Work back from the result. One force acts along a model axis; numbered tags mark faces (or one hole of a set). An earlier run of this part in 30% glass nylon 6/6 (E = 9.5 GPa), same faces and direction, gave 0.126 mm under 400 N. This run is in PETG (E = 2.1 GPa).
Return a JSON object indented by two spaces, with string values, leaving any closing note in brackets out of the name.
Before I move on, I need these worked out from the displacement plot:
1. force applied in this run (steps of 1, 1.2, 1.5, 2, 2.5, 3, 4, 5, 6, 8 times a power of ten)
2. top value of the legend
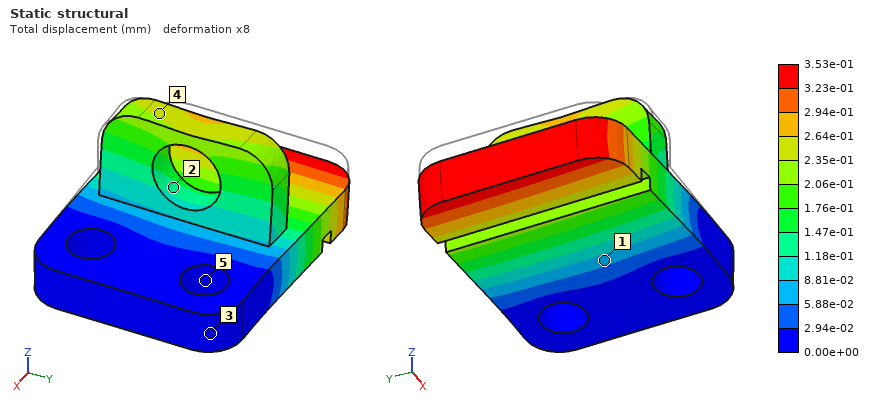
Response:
{
  "force applied in this run": "250 N",
  "top value of the legend": "3.53e-01 mm"
}
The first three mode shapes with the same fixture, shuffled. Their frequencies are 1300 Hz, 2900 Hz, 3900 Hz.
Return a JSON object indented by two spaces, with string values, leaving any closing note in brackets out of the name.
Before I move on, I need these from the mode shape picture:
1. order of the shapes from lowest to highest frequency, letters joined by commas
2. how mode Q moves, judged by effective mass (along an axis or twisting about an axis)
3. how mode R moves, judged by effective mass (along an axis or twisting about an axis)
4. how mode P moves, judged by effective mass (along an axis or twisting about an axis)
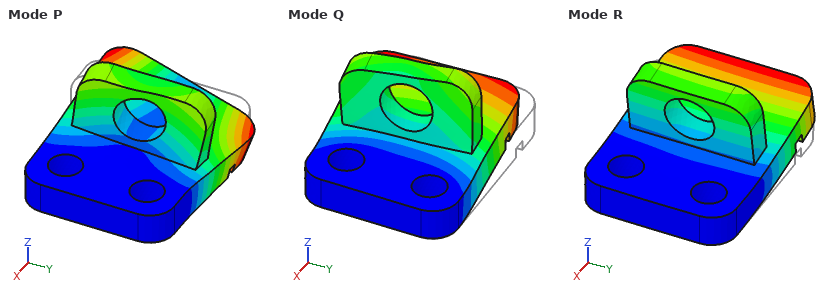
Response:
{
  "order of the shapes from lowest to highest frequency, letters joined by commas": "R, P, Q",
  "how mode Q moves, judged by effective mass": "along Y",
  "how mode R moves, judged by effective mass": "along Z",
  "how mode P moves, judged by effective mass": "twisting about X"
}
